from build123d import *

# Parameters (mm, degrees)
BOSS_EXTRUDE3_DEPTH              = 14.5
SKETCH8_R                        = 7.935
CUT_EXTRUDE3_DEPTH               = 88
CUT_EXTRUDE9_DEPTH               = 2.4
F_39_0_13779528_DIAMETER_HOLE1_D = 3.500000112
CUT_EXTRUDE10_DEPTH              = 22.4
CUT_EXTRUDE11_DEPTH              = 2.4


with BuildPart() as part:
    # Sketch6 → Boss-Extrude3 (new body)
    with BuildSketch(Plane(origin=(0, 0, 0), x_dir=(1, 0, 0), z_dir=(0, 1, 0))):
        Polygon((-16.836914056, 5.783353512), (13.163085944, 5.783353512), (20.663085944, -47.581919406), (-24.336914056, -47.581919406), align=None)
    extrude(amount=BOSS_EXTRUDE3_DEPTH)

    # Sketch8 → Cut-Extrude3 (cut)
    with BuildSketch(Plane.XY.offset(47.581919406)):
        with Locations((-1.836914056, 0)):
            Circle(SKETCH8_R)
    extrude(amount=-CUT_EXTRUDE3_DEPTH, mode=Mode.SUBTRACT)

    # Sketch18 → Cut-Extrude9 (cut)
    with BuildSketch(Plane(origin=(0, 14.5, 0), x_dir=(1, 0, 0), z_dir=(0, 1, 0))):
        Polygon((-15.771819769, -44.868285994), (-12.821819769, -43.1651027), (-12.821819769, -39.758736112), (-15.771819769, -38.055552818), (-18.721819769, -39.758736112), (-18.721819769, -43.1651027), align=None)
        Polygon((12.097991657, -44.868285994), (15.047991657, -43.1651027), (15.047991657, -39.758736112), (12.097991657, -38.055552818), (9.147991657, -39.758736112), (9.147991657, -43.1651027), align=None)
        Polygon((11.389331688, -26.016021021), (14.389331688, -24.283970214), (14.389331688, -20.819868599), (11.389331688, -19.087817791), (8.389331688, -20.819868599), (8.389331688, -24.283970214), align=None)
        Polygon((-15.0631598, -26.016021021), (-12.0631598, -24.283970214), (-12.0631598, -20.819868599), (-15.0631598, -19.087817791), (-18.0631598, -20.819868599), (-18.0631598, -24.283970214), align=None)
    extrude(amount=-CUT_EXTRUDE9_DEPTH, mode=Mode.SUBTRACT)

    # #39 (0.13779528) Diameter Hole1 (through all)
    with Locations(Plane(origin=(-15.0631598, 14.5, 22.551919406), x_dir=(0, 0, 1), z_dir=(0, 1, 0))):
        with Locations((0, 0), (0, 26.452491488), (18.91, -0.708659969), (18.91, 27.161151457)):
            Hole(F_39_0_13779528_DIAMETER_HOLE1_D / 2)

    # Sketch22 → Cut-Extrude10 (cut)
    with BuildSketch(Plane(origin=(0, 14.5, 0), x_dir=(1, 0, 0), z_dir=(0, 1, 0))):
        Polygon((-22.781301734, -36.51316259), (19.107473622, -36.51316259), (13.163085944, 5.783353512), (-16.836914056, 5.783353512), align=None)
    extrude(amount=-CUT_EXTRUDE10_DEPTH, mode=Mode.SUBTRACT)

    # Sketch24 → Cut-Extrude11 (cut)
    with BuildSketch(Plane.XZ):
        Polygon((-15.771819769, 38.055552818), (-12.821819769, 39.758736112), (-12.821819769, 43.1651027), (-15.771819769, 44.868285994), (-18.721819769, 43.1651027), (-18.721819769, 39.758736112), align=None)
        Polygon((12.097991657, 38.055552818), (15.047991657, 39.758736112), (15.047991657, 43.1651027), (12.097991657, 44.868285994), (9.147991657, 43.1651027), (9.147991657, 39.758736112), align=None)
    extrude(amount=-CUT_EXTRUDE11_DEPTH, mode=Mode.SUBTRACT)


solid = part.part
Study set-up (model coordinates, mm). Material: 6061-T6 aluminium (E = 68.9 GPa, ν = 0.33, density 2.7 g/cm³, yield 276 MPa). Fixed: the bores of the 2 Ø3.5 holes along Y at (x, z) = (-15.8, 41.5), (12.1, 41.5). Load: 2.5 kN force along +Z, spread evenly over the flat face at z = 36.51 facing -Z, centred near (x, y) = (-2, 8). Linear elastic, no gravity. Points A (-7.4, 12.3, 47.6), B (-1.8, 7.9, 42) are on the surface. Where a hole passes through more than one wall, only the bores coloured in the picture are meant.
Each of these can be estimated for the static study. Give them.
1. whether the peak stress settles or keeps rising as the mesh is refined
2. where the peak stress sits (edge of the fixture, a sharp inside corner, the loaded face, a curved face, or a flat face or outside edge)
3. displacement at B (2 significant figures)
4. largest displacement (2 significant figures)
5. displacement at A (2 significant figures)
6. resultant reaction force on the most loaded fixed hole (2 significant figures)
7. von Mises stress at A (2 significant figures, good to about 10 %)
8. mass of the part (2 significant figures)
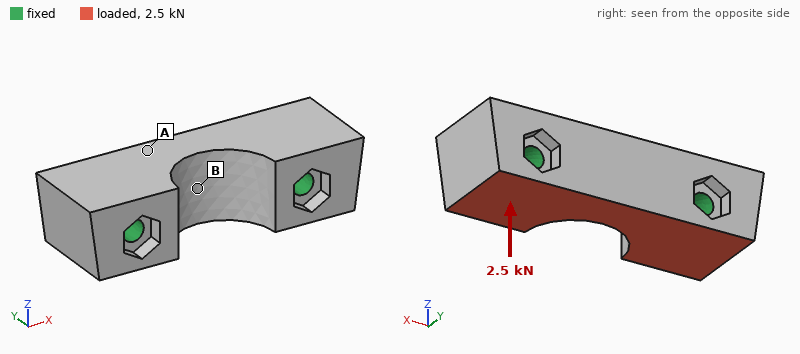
keeps rising
edge of the fixture
2.9 µm
4.2 µm
2.9 µm
1.3 kN
6.9 MPa
15 g
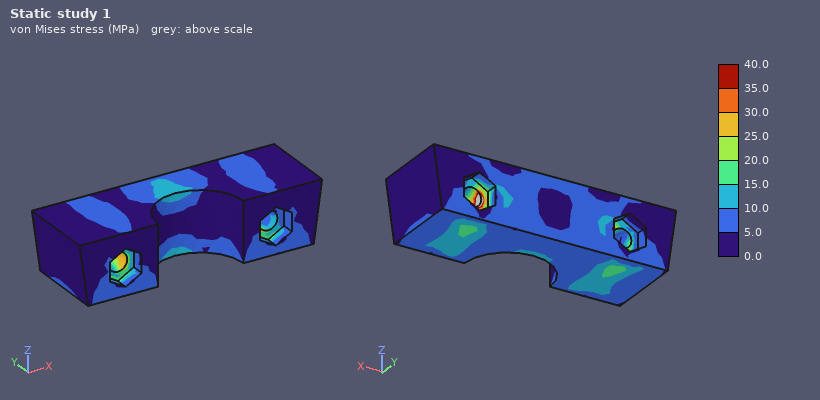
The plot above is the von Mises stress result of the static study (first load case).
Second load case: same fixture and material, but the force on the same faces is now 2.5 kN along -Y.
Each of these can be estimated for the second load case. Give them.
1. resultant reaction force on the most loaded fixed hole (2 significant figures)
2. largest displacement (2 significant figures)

1.3 kN
7.5 µm
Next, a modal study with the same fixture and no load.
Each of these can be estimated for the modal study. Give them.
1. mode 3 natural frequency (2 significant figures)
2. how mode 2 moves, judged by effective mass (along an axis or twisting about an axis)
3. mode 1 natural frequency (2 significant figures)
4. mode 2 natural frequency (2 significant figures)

51 kHz
along Y
34 kHz
44 kHz
